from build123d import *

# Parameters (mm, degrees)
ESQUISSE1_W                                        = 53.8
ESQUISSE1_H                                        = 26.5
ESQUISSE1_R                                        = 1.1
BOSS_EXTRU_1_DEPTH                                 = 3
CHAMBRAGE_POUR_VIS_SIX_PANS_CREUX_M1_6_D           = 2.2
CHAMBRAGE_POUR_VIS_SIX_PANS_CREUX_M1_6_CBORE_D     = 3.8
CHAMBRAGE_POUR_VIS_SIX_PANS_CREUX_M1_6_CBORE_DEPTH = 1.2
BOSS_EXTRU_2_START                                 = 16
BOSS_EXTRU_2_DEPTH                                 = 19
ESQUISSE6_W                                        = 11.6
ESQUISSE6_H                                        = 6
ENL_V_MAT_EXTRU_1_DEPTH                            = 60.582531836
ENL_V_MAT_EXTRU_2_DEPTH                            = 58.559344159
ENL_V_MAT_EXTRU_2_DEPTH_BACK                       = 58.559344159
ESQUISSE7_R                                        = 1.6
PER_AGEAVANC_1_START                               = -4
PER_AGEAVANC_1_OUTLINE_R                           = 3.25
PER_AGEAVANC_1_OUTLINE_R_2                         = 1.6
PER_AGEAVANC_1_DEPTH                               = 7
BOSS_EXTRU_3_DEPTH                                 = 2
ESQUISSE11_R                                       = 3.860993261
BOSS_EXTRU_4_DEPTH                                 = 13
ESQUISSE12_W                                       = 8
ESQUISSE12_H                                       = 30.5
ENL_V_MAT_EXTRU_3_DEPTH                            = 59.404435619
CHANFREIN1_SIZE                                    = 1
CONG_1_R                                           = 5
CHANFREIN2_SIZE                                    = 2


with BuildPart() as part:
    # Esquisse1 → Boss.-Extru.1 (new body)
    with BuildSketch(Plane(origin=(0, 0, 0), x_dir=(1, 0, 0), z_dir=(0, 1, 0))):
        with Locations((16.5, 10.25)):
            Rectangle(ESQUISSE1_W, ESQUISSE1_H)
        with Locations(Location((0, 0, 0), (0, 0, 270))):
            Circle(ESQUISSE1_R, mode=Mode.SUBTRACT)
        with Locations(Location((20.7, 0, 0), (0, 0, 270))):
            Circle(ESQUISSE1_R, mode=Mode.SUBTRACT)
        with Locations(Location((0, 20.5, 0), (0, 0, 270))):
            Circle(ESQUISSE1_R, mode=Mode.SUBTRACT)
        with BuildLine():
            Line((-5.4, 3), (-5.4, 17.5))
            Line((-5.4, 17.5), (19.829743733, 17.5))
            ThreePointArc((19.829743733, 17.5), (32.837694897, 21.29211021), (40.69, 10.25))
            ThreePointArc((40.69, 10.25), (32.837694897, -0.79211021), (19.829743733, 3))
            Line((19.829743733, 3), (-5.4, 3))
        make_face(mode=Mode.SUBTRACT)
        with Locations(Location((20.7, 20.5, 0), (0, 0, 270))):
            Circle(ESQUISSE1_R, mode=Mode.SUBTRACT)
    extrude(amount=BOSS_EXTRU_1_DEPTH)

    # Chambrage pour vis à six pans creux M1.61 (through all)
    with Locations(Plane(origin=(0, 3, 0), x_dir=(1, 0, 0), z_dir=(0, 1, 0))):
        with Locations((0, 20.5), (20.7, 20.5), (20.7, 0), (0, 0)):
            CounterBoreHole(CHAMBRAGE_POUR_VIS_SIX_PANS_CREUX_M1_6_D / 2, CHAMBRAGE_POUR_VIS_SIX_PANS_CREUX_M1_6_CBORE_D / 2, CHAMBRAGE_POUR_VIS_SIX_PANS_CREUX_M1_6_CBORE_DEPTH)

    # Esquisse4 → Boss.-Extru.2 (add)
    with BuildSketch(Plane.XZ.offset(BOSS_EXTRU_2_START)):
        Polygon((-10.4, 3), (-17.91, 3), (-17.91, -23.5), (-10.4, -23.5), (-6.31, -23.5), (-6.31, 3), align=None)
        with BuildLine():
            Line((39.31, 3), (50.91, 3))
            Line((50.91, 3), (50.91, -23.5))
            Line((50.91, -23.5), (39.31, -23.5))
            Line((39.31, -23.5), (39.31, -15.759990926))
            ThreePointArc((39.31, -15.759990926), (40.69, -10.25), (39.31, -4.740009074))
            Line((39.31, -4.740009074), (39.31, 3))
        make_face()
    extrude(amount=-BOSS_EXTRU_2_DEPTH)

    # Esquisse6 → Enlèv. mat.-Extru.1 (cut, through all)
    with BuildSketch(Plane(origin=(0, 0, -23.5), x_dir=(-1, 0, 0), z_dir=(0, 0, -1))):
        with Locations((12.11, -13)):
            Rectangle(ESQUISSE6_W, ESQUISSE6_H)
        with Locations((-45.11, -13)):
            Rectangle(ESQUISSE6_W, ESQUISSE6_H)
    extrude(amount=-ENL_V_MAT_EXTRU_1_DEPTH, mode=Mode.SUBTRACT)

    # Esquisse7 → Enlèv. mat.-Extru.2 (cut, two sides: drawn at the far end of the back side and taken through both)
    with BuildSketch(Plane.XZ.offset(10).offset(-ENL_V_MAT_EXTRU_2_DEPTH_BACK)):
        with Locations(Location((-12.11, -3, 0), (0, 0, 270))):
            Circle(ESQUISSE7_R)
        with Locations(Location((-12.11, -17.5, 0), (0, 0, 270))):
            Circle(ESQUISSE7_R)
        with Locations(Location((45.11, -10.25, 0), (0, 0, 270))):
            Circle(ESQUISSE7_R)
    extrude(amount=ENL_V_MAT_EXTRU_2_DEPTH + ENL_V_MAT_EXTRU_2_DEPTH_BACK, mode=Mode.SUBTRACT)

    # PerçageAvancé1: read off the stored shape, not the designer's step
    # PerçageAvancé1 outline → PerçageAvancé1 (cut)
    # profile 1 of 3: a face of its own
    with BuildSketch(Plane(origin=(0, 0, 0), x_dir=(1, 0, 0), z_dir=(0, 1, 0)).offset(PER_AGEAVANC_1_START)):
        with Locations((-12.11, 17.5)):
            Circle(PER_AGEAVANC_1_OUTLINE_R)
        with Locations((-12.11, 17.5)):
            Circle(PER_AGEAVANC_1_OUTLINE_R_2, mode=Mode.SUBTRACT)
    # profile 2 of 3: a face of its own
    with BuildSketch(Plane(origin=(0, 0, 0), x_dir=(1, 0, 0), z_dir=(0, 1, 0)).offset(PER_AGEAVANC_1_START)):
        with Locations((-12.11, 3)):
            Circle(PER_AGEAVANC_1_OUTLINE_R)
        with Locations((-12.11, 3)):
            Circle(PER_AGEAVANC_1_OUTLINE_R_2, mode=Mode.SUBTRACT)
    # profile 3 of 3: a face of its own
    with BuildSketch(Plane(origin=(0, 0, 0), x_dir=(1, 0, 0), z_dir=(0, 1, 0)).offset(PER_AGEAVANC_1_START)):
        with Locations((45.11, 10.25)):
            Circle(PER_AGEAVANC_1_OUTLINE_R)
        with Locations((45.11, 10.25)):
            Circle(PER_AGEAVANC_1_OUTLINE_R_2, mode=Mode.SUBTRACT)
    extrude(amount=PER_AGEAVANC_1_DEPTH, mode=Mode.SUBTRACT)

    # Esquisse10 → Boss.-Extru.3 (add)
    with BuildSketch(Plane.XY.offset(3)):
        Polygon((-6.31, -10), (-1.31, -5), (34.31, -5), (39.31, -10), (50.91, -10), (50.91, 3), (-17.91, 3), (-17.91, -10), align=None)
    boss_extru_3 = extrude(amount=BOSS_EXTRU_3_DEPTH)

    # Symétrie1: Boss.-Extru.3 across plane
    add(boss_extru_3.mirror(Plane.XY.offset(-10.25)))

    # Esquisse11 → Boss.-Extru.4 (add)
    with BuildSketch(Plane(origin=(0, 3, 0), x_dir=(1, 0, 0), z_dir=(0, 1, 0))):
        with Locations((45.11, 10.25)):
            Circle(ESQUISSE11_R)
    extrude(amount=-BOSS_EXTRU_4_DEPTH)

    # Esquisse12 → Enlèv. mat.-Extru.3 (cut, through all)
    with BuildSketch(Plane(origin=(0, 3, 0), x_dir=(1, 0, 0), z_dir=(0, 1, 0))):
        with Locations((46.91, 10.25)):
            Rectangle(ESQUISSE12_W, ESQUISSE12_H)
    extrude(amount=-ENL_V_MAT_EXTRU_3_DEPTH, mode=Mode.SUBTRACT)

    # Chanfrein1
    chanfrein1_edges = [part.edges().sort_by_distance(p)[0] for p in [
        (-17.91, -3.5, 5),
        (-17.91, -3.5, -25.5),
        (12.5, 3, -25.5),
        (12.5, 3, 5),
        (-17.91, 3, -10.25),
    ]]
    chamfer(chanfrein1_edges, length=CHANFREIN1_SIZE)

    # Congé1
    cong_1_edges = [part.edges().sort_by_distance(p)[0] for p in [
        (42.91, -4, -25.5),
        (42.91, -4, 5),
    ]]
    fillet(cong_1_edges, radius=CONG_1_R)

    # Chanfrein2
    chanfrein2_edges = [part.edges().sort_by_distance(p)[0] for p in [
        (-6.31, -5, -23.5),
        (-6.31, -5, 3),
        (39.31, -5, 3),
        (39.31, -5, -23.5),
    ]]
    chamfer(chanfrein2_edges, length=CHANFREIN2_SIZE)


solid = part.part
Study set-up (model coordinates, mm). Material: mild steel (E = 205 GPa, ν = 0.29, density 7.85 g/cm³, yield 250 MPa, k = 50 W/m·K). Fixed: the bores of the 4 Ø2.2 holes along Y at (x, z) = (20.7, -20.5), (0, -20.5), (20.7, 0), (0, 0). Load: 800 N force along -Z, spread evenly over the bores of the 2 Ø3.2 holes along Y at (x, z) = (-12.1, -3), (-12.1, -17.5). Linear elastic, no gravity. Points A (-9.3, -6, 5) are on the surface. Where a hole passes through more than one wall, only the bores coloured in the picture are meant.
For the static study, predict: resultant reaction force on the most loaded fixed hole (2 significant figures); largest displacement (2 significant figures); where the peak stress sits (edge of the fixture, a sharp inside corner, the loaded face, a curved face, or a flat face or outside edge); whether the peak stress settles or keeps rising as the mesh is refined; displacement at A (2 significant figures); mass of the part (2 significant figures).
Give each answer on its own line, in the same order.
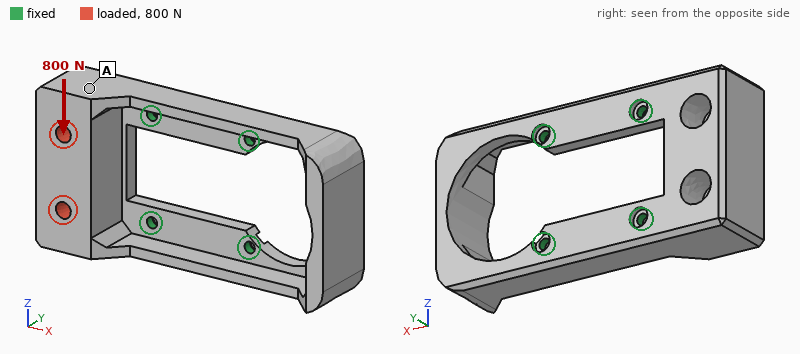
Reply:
550 N
9.4 µm
edge of the fixture
keeps rising
7.6 µm
63 g
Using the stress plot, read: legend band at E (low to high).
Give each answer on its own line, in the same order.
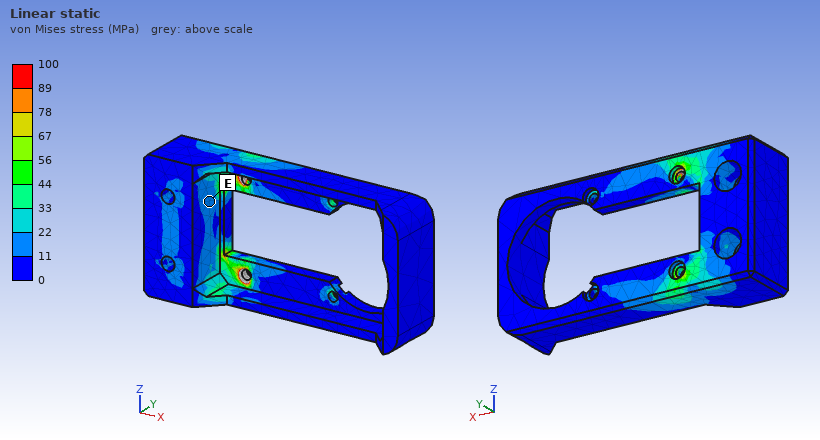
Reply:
11 to 22 MPa
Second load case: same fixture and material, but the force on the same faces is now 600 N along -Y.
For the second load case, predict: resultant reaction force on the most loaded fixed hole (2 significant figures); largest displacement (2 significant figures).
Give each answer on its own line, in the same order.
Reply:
450 N
29 µm
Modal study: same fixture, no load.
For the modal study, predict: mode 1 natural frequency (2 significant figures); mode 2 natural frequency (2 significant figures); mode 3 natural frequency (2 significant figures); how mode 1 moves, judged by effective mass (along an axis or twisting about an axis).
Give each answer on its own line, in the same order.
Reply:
3800 Hz
4600 Hz
4600 Hz
along Y
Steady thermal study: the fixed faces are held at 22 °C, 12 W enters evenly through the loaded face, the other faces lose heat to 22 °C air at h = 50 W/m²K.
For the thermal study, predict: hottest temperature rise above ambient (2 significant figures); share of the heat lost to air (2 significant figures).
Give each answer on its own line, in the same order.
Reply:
36 K
29 %
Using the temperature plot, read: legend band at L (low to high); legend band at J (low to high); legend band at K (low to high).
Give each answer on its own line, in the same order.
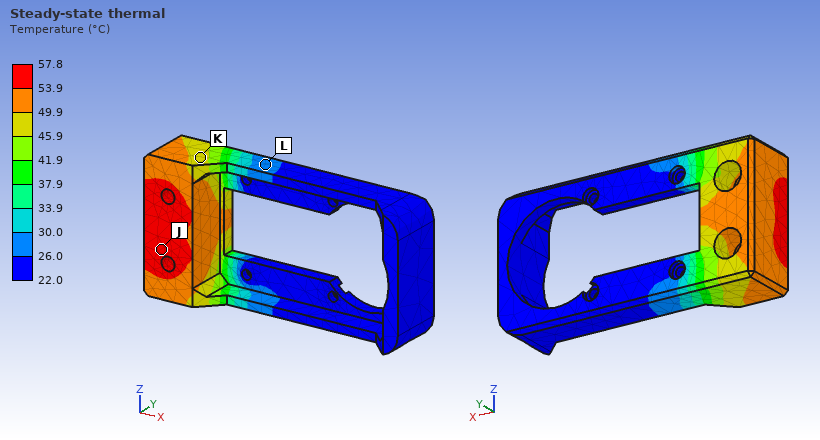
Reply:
26.0 to 30.0 °C
53.9 to 57.8 °C
45.9 to 49.9 °C
